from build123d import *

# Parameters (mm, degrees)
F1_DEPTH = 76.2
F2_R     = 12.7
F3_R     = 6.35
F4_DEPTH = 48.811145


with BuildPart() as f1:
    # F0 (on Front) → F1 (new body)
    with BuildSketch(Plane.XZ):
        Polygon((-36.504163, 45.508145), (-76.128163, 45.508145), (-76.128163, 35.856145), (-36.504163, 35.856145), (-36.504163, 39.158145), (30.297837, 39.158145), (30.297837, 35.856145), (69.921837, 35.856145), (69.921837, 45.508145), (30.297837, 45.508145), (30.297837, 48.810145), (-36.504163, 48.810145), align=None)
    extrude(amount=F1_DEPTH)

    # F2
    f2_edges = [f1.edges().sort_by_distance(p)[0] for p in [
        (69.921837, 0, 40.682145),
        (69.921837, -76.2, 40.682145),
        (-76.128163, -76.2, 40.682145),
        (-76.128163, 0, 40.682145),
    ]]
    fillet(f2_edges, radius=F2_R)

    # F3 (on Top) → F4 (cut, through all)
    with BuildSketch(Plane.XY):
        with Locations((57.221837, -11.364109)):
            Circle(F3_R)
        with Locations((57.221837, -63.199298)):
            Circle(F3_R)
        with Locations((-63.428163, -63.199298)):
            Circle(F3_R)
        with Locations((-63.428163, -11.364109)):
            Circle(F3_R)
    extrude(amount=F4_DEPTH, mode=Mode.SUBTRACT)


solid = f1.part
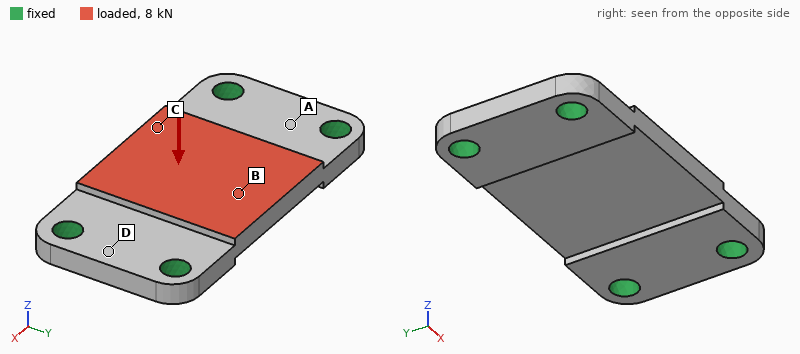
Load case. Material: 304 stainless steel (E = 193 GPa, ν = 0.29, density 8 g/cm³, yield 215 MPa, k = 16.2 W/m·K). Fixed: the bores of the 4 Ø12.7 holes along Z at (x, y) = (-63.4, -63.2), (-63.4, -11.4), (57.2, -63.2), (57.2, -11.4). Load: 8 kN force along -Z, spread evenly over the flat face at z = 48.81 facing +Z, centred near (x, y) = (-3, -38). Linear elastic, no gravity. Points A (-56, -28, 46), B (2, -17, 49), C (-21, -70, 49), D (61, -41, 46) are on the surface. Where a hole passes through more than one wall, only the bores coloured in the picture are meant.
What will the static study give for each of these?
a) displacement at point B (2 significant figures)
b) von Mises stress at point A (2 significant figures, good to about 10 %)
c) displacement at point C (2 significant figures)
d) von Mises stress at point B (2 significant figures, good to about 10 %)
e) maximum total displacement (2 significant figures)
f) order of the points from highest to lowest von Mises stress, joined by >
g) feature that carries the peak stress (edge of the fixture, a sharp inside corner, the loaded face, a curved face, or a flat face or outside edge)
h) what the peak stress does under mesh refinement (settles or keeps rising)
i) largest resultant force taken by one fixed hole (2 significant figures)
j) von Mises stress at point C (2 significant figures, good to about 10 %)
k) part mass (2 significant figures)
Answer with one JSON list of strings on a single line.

["38 µm", "25 MPa", "32 µm", "49 MPa", "41 µm", "B > C > A > D", "edge of the fixture", "keeps rising", "4.0 kN", "38 MPa", "810 g"]
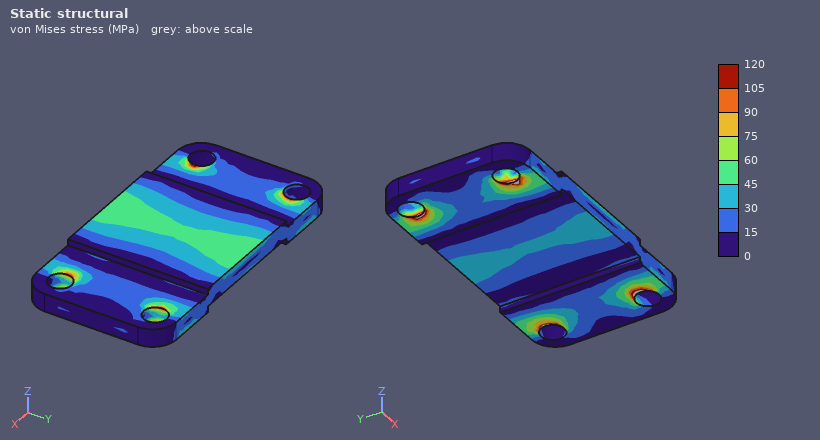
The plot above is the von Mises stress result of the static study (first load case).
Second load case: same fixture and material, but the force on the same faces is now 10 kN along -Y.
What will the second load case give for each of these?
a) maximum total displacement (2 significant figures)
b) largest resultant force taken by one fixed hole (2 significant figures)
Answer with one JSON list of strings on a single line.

["16 µm", "3.7 kN"]
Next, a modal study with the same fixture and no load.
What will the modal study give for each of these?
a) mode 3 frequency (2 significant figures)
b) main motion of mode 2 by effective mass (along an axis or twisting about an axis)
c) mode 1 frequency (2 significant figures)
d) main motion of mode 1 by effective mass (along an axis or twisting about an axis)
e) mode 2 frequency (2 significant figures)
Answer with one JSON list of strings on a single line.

["8600 Hz", "twisting about X", "3800 Hz", "along Z", "5200 Hz"]
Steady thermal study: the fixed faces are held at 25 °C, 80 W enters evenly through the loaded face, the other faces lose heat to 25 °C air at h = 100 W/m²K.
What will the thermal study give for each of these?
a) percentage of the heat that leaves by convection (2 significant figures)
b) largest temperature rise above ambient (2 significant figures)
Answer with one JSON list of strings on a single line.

["68 %", "74 K"]
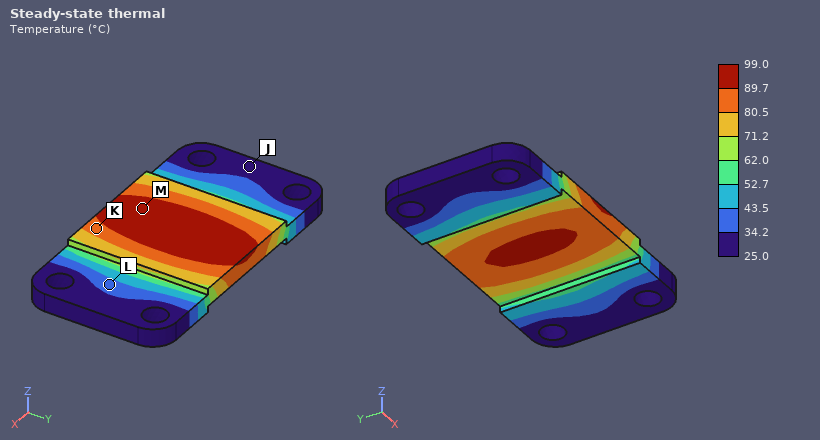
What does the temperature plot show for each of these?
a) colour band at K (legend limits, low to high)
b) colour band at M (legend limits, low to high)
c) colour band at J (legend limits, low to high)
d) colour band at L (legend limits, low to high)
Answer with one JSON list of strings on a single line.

["80.5 to 89.7 °C", "89.7 to 99.0 °C", "25.0 to 34.2 °C", "34.2 to 43.5 °C"]
